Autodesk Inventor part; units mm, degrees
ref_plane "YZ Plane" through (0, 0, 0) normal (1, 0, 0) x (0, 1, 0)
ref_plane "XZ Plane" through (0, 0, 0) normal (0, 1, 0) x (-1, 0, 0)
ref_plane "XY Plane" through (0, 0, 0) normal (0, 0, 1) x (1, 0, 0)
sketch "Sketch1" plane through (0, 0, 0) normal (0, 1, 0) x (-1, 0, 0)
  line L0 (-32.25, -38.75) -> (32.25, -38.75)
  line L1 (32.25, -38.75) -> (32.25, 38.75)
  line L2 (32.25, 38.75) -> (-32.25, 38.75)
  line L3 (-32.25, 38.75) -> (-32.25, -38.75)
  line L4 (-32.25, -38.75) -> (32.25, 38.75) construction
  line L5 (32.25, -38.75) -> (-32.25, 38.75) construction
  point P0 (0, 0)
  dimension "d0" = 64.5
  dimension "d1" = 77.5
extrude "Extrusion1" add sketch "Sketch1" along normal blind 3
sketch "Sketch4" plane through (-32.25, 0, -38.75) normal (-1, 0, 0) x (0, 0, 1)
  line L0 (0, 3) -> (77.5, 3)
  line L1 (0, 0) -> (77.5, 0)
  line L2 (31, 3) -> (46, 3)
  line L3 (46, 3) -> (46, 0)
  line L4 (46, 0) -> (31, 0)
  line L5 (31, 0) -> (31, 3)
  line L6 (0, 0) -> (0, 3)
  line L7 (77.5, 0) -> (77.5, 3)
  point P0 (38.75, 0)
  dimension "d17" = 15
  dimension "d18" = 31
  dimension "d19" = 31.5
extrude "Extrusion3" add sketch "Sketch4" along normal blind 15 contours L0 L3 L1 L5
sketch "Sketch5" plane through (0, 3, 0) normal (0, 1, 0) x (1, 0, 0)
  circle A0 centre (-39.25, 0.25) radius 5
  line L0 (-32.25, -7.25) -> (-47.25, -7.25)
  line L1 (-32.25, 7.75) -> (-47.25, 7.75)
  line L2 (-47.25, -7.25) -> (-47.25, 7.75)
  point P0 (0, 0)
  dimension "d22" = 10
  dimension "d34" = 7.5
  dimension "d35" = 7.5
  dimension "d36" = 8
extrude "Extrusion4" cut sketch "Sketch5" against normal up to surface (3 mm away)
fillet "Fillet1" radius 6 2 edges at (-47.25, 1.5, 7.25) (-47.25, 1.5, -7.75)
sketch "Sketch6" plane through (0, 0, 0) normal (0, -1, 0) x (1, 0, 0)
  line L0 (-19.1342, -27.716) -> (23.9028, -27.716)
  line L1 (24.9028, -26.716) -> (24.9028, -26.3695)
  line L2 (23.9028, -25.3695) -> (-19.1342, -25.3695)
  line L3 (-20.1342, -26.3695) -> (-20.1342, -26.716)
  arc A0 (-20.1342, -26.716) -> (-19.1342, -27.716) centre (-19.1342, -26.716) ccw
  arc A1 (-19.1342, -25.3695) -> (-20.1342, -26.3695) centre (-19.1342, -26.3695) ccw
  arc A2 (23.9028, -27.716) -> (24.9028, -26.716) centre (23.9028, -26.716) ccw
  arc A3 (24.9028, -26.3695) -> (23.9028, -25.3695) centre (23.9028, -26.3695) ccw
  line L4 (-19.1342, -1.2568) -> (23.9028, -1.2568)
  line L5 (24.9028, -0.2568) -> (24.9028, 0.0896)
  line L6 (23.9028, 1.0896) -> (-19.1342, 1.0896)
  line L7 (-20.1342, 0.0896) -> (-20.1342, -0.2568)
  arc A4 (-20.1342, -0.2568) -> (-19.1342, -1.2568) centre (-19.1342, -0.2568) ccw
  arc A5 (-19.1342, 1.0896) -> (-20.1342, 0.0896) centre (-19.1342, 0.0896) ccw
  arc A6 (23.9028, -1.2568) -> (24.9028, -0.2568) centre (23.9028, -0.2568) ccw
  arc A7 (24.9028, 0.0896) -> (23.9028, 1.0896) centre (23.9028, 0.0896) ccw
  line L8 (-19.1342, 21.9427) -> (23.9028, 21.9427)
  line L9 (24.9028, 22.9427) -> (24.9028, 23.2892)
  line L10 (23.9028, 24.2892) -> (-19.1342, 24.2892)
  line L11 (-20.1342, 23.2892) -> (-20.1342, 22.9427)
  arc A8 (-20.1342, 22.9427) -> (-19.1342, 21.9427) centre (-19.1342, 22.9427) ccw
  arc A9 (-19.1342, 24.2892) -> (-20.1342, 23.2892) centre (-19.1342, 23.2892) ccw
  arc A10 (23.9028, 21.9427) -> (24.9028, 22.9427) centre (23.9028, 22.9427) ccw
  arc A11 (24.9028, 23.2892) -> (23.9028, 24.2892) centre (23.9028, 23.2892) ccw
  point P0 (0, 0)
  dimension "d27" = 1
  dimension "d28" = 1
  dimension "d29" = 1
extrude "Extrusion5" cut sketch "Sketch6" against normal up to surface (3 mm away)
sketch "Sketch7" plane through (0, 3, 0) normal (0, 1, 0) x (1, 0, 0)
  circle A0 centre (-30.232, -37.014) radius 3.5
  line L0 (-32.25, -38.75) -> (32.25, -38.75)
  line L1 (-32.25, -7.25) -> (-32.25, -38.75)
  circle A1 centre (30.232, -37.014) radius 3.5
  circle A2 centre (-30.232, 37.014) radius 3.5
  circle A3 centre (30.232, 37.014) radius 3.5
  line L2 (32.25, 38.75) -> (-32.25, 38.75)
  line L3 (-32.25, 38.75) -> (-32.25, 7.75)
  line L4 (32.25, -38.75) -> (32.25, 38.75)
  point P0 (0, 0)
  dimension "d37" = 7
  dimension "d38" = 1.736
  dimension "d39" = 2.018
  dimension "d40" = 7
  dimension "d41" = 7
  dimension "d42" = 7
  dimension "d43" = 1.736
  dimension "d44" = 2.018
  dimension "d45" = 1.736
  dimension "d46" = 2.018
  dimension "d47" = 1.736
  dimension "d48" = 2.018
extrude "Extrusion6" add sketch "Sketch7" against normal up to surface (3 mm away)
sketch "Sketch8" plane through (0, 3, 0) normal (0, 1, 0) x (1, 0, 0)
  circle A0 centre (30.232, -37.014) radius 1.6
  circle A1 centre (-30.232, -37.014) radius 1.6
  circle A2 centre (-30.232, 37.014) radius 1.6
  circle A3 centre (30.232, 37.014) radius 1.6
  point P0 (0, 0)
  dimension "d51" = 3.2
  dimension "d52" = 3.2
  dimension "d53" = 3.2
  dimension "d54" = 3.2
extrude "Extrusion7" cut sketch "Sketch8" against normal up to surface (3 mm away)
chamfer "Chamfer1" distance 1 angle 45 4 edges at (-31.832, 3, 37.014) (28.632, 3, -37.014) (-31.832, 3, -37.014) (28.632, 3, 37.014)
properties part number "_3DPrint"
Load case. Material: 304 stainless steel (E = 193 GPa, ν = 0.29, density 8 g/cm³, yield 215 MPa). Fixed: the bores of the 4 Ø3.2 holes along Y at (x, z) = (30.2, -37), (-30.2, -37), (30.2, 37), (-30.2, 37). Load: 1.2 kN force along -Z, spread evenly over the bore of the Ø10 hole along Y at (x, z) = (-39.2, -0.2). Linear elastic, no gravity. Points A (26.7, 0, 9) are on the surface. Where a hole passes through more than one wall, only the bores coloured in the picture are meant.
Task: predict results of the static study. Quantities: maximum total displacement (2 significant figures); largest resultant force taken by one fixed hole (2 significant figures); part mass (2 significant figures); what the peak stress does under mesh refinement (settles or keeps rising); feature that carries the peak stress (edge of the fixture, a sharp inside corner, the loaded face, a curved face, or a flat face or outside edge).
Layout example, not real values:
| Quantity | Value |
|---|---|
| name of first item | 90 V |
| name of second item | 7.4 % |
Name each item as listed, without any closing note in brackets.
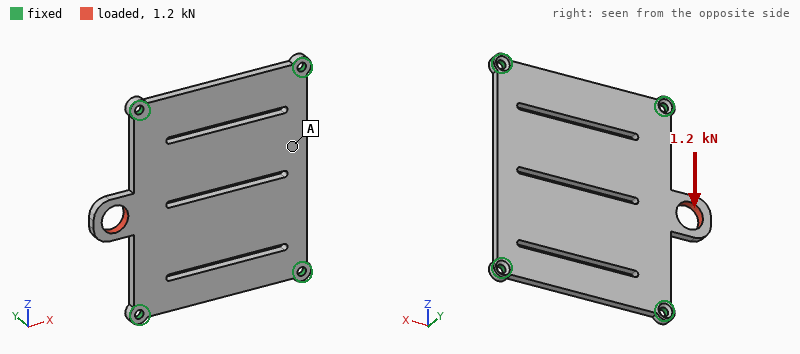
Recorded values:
| Quantity | Value |
|---|---|
| maximum total displacement | 41 µm |
| largest resultant force taken by one fixed hole | 550 N |
| part mass | 120 g |
| what the peak stress does under mesh refinement | keeps rising |
| feature that carries the peak stress | a sharp inside corner |
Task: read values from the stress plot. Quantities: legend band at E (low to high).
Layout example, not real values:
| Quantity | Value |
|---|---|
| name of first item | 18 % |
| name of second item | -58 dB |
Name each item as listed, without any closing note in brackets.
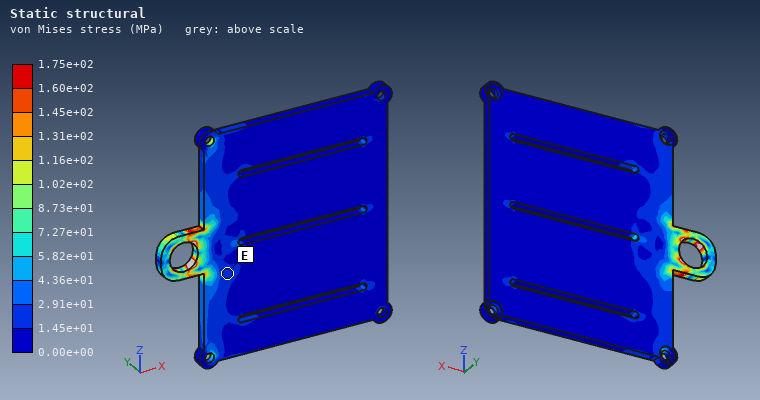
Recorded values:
| Quantity | Value |
|---|---|
| legend band at E | 1.45e+01 to 2.91e+01 MPa |
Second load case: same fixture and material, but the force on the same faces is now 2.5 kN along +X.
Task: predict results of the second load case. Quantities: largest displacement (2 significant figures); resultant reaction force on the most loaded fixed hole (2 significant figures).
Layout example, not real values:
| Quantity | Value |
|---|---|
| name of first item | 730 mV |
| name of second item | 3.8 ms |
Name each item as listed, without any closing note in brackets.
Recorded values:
| Quantity | Value |
|---|---|
| largest displacement | 26 µm |
| resultant reaction force on the most loaded fixed hole | 790 N |
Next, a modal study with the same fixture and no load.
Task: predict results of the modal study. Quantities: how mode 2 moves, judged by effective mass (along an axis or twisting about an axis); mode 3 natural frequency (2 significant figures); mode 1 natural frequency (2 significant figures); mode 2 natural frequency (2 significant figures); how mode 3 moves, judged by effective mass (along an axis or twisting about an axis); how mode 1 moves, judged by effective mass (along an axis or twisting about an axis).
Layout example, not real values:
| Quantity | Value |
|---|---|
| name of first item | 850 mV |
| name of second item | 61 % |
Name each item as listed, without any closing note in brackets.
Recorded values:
| Quantity | Value |
|---|---|
| how mode 2 moves, judged by effective mass | twisting about Z |
| mode 3 natural frequency | 3100 Hz |
| mode 1 natural frequency | 1500 Hz |
| mode 2 natural frequency | 2600 Hz |
| how mode 3 moves, judged by effective mass | twisting about X |
| how mode 1 moves, judged by effective mass | along Y |
